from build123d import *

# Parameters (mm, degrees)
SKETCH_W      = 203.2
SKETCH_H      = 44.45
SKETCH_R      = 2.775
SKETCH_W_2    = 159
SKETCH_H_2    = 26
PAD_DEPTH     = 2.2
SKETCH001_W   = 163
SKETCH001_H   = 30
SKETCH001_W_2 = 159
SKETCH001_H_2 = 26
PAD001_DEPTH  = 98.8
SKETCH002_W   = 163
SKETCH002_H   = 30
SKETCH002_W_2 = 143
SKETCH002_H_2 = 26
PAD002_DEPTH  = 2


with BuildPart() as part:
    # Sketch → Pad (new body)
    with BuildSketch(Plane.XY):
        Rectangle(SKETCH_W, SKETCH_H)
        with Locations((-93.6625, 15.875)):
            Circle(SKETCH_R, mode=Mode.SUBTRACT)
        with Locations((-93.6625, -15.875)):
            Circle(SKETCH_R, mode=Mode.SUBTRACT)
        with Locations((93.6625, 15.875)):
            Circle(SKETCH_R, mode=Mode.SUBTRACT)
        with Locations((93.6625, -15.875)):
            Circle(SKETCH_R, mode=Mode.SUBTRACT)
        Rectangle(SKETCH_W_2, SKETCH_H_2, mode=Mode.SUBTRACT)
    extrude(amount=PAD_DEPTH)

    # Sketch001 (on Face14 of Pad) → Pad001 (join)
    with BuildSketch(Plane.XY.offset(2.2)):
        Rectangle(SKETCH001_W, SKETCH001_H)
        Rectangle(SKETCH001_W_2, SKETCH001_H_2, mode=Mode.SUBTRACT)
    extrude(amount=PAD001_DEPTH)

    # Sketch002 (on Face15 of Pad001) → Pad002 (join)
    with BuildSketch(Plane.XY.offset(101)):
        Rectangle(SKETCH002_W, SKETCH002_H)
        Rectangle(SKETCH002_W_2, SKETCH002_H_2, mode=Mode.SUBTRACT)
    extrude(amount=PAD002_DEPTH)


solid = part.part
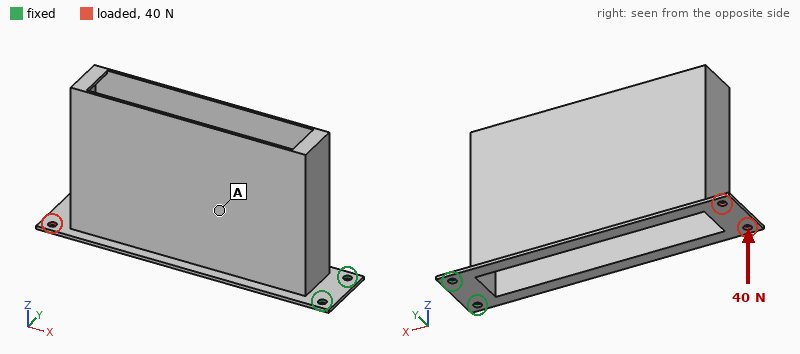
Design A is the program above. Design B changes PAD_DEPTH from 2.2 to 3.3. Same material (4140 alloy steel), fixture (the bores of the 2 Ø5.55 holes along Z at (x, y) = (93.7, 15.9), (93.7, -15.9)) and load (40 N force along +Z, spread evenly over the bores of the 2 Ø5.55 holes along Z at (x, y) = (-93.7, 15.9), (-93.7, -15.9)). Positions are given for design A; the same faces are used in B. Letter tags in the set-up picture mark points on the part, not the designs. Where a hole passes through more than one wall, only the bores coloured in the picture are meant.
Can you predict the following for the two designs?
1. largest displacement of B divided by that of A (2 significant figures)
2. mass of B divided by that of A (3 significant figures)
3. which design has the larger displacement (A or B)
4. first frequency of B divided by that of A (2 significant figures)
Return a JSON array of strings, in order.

["0.37", "1.05", "A", "1.6"]
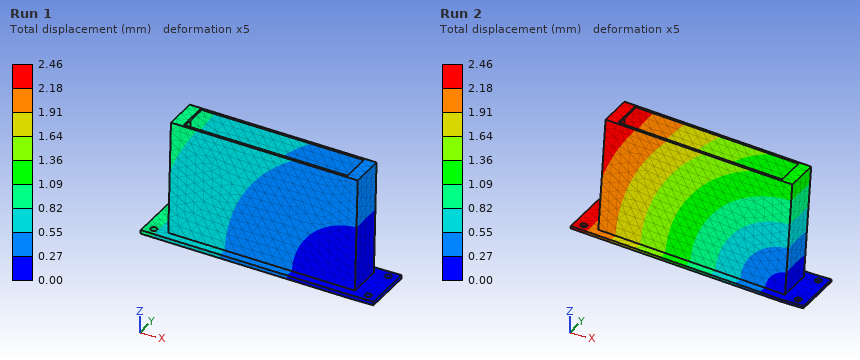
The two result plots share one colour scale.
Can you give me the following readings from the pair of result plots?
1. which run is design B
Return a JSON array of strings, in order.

["Run 1"]
